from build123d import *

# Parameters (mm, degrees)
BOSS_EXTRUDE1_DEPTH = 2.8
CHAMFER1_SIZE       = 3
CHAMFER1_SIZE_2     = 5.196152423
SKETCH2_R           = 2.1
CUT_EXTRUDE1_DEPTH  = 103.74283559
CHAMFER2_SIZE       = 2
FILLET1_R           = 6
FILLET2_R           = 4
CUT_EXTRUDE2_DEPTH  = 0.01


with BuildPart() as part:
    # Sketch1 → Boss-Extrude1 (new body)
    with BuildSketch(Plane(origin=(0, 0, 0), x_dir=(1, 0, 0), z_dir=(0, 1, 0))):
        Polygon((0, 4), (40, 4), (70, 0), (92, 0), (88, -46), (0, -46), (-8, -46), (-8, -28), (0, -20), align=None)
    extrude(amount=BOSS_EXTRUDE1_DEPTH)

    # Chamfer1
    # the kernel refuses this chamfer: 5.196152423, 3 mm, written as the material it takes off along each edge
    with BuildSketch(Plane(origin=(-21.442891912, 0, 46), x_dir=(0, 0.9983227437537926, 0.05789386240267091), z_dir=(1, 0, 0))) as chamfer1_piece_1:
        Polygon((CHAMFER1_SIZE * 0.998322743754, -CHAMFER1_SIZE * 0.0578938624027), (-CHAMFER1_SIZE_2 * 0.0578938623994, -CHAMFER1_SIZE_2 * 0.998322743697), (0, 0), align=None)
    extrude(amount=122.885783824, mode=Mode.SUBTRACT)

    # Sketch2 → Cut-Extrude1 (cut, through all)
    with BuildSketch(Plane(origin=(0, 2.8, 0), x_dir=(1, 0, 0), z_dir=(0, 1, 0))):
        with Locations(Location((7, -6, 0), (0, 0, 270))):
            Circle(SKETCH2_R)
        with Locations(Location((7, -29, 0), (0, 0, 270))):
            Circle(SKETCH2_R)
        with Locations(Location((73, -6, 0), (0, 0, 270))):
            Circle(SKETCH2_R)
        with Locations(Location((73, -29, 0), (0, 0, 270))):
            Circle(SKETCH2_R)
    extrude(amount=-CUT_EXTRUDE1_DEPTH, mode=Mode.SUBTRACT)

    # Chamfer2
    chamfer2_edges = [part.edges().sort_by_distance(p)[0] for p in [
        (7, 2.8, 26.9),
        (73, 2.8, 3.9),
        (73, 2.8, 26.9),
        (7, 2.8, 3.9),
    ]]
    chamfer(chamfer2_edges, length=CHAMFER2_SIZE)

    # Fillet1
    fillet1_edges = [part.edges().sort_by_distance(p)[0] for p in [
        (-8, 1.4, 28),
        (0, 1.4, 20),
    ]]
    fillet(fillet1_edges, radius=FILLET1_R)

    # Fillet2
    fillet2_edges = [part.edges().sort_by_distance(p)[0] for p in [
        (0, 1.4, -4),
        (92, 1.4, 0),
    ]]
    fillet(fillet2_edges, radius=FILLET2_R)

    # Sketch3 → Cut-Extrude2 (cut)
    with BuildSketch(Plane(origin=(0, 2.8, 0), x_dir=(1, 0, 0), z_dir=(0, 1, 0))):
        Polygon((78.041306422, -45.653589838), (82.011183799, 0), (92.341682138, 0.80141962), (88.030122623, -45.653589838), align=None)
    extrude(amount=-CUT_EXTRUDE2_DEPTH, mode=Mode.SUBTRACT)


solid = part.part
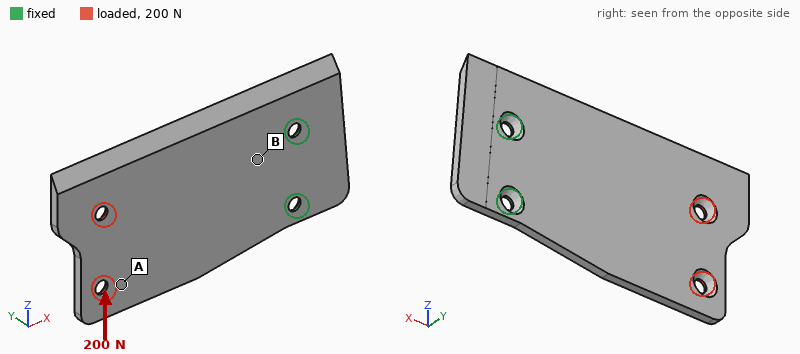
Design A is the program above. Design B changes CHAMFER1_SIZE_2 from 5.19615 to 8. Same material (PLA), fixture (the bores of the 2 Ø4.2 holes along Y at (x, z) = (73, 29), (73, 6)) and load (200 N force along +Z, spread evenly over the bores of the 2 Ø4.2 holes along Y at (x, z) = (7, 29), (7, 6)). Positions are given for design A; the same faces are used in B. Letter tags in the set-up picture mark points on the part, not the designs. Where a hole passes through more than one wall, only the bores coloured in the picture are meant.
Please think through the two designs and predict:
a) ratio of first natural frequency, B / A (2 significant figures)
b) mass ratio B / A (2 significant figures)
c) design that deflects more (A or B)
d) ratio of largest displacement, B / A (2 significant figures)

1.0
0.97
B
1.1
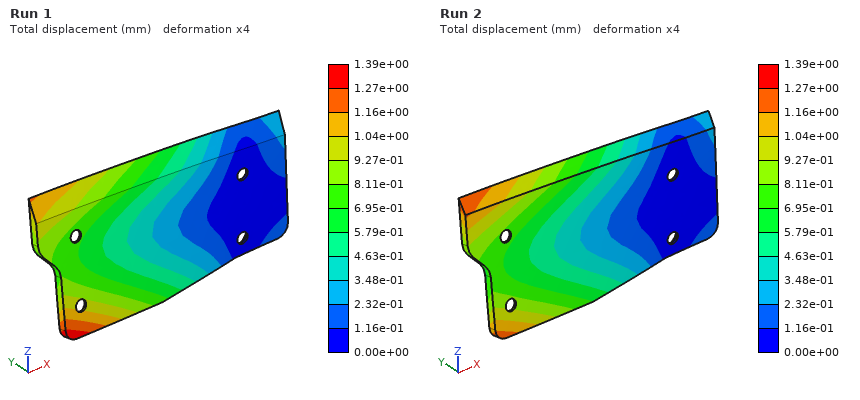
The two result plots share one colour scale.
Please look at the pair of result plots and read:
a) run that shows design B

Run 1
